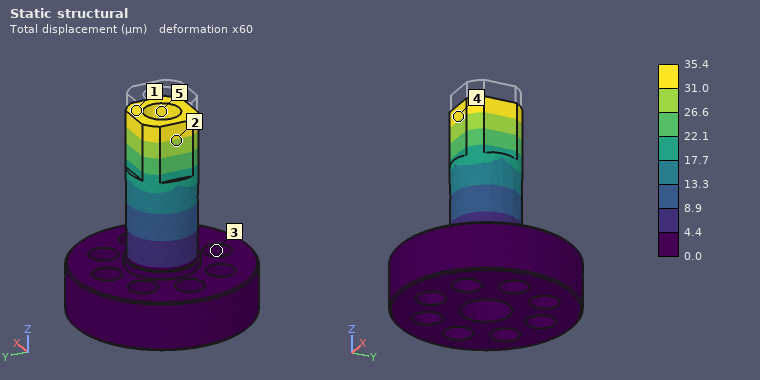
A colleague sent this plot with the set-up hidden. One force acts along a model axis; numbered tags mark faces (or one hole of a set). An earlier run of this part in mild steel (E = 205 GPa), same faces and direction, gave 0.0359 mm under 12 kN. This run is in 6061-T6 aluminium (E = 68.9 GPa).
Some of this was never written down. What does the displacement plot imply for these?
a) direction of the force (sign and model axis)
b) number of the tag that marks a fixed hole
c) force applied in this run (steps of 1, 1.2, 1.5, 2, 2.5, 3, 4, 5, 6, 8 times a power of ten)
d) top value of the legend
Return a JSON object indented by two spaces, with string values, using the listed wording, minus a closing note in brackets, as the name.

{
  "direction of the force": "-Z",
  "number of the tag that marks a fixed hole": "3",
  "force applied in this run": "4 kN",
  "top value of the legend": "35.4 µm"
}
